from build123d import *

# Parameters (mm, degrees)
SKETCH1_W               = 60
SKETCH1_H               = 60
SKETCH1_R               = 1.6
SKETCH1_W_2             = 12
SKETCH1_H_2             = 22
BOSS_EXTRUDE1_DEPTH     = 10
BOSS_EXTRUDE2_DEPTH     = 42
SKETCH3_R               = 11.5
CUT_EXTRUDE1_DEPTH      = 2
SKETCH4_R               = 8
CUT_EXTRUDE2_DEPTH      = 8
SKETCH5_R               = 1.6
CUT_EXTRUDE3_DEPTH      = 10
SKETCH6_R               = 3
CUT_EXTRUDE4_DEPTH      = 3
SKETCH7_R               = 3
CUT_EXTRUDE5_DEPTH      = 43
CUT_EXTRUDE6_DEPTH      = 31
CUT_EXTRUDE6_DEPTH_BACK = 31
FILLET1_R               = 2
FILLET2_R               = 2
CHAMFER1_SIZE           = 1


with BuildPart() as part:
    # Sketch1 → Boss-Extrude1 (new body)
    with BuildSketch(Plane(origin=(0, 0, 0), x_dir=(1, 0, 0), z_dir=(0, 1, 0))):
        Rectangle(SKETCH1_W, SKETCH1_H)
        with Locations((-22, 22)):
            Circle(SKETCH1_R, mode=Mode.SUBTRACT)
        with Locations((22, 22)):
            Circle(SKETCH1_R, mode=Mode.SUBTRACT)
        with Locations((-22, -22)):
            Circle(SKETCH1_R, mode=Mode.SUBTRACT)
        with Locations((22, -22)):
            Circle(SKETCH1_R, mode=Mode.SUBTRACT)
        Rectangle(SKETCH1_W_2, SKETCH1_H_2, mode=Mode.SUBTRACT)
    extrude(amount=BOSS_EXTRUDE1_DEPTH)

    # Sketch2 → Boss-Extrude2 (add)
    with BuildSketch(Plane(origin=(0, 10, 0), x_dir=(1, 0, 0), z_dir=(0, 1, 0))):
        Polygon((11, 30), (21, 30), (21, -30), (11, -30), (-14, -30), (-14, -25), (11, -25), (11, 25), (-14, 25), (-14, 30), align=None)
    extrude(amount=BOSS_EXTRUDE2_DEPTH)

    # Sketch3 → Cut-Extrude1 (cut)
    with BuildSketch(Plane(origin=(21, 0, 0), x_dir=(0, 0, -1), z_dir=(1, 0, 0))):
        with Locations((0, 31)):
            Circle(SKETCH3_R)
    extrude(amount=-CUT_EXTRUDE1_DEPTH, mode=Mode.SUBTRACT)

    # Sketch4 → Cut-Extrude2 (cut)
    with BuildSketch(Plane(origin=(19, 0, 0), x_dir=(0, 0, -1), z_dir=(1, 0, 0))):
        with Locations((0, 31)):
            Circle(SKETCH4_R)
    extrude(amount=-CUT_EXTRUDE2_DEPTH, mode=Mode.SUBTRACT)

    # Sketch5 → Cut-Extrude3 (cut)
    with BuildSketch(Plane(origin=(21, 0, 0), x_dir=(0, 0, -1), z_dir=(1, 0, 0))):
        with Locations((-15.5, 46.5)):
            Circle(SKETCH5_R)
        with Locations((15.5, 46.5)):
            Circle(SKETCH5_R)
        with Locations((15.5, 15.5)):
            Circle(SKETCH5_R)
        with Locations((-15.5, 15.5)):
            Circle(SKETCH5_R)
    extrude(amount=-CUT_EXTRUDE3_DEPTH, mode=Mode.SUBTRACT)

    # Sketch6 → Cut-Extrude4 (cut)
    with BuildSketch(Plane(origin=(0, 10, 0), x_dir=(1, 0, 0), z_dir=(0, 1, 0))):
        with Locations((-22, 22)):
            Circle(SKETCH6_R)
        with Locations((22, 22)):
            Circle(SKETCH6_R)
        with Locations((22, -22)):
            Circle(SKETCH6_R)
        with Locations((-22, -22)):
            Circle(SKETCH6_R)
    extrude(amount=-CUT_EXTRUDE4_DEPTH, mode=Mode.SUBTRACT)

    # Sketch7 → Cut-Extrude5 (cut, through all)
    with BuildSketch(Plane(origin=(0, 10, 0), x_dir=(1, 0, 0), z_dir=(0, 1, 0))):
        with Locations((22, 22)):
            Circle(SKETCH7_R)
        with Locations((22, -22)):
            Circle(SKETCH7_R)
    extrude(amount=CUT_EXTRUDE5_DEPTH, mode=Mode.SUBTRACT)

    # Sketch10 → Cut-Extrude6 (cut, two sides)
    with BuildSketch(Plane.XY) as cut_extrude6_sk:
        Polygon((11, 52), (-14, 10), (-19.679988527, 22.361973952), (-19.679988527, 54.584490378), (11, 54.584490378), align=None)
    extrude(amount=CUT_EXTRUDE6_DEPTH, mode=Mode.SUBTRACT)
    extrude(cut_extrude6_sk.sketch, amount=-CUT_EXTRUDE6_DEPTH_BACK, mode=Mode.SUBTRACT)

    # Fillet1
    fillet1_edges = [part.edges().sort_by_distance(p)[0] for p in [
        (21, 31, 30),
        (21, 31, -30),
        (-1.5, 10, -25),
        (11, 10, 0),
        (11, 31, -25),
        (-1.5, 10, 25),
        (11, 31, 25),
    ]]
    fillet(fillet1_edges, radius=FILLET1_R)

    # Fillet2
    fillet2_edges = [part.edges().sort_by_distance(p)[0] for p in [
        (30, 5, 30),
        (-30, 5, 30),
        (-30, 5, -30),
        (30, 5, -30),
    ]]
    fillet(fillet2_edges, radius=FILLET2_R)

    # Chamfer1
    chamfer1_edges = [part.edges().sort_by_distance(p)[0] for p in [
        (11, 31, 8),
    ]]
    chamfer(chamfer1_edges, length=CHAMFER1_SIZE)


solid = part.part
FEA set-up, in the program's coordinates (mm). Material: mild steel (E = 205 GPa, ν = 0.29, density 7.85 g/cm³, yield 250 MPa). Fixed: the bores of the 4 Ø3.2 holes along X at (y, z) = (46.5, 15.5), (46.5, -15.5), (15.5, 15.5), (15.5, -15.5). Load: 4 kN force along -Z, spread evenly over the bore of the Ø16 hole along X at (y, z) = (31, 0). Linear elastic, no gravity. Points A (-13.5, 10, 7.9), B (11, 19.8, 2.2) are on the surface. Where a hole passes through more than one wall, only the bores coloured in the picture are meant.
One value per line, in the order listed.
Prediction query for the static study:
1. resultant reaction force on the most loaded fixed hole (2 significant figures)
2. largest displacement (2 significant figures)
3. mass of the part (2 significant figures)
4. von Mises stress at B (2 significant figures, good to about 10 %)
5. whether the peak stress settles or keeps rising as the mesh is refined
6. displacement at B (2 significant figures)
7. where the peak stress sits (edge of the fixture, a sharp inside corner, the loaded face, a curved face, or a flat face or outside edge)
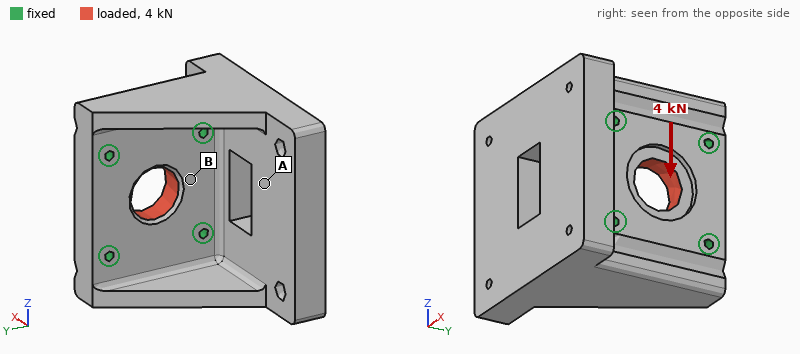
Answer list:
1.0 kN
0.94 µm
470 g
7.7 MPa
keeps rising
0.45 µm
edge of the fixture
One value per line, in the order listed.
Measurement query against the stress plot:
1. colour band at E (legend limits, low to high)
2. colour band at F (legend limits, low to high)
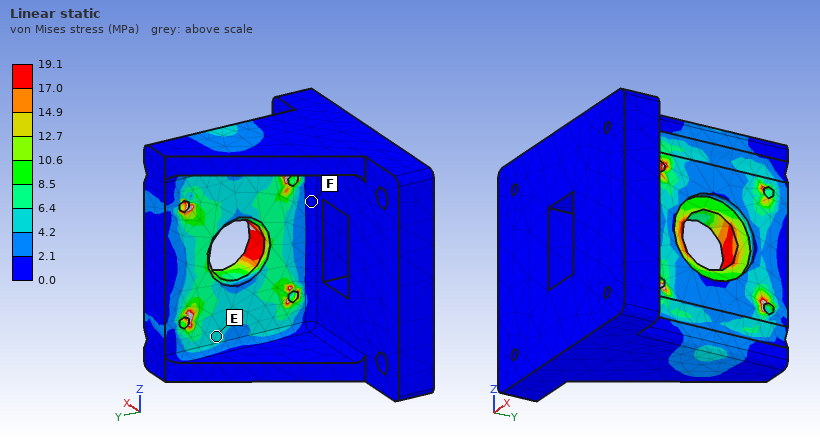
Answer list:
4.2 to 6.4 MPa
0.0 to 2.1 MPa
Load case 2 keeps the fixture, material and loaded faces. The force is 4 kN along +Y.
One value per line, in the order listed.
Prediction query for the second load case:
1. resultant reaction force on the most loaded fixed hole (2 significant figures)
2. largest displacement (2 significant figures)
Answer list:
1.1 kN
1.2 µm
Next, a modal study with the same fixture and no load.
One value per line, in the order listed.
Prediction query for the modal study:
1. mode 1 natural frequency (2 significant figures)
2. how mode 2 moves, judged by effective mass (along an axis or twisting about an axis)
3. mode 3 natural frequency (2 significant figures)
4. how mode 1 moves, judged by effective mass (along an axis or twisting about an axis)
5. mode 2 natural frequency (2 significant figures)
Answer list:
4600 Hz
along Z
10000 Hz
along Y
5800 Hz
